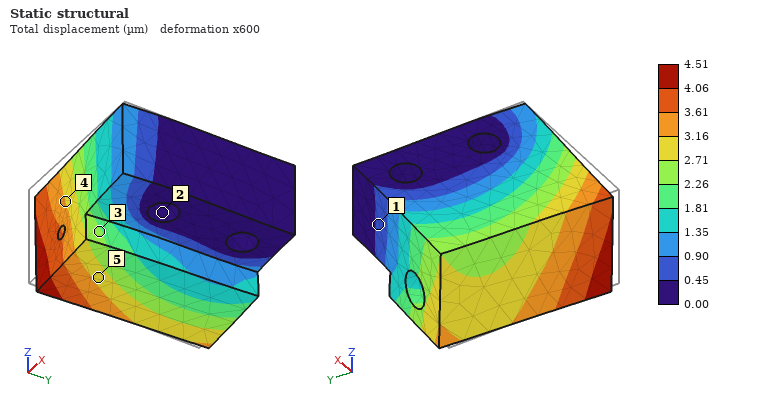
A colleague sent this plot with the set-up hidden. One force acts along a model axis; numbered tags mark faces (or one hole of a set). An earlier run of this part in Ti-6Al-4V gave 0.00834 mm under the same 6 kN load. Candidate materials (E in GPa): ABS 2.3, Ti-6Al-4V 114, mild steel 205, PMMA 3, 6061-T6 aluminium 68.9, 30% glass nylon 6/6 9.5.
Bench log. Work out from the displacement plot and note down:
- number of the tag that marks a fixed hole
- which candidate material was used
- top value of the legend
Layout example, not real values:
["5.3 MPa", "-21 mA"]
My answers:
["2", "mild steel", "4.51 µm"]
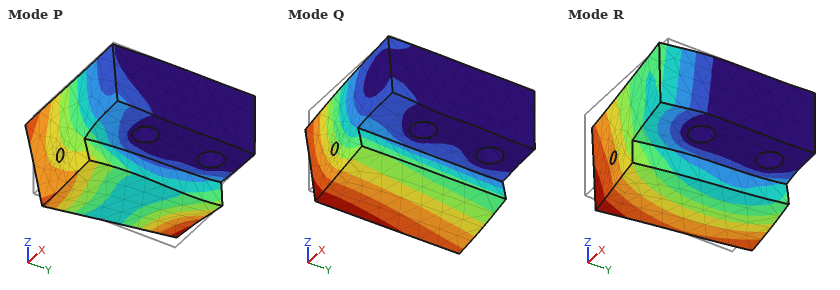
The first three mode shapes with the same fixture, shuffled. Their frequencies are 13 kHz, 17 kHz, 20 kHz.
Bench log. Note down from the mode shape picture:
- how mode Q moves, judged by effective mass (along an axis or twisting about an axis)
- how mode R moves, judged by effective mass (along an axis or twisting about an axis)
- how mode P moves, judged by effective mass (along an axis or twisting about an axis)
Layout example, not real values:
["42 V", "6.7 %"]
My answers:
["along Z", "along Y", "twisting about X"]
